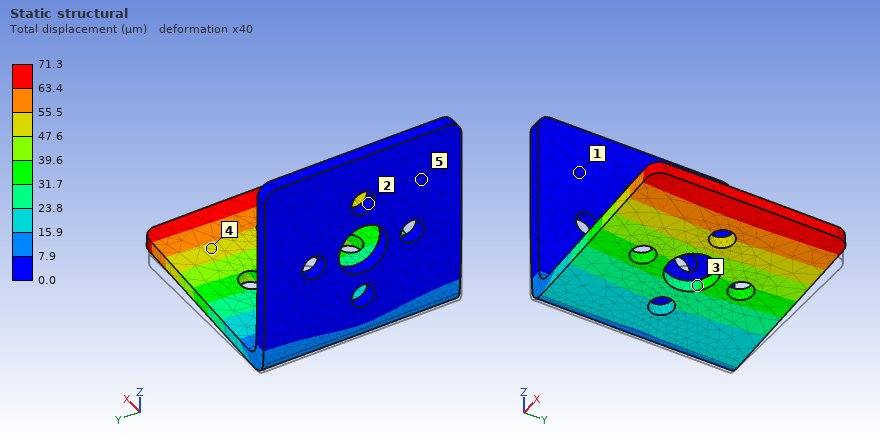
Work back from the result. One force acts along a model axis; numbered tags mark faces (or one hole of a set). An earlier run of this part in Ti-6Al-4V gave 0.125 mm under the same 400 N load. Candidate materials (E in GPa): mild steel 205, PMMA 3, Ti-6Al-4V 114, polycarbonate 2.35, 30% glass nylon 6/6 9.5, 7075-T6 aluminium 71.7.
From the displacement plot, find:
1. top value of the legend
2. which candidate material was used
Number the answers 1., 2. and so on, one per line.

1. 71.3 µm
2. mild steel
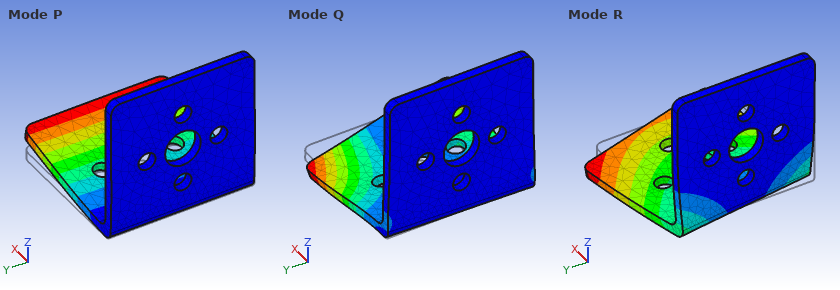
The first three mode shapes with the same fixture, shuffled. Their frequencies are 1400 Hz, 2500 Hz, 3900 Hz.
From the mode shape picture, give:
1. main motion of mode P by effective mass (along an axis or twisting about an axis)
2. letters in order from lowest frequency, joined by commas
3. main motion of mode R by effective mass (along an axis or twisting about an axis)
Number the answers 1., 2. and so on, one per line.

1. along Z
2. P, R, Q
3. along Y
